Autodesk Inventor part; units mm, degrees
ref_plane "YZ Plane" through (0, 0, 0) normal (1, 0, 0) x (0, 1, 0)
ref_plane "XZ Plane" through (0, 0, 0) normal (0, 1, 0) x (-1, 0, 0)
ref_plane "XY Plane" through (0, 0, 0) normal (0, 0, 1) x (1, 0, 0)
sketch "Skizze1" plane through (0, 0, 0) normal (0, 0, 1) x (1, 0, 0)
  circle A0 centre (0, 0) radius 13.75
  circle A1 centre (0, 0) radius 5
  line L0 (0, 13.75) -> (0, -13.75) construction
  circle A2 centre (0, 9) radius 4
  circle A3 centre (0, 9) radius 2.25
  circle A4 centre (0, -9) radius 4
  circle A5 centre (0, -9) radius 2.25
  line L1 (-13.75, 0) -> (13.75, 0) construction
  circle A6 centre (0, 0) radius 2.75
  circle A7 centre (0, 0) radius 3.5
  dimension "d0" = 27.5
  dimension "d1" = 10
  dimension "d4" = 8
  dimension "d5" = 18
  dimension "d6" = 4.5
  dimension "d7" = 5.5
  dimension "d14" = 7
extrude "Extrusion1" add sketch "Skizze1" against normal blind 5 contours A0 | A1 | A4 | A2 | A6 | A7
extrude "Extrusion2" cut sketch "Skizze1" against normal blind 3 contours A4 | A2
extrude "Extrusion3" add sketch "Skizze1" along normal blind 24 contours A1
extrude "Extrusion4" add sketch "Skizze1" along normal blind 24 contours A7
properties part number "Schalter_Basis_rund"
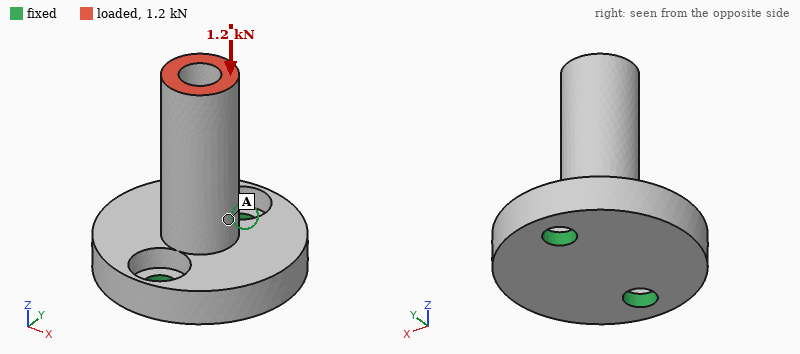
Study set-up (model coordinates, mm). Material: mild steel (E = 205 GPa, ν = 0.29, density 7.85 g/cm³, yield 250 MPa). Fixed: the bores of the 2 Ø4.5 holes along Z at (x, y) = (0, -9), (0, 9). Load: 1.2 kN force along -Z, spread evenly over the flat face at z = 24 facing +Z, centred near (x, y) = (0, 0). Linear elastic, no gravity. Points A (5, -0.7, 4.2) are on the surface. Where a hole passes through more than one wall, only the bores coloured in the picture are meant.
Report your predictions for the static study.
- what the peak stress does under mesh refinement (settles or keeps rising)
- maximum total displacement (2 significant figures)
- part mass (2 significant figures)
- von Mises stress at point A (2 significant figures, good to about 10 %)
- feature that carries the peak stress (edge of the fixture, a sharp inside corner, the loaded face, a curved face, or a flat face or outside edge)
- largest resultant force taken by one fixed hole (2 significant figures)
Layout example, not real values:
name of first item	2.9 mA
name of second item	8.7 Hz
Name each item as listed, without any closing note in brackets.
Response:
what the peak stress does under mesh refinement	keeps rising
maximum total displacement	4.7 µm
part mass	31 g
von Mises stress at point A	19 MPa
feature that carries the peak stress	edge of the fixture
largest resultant force taken by one fixed hole	660 N
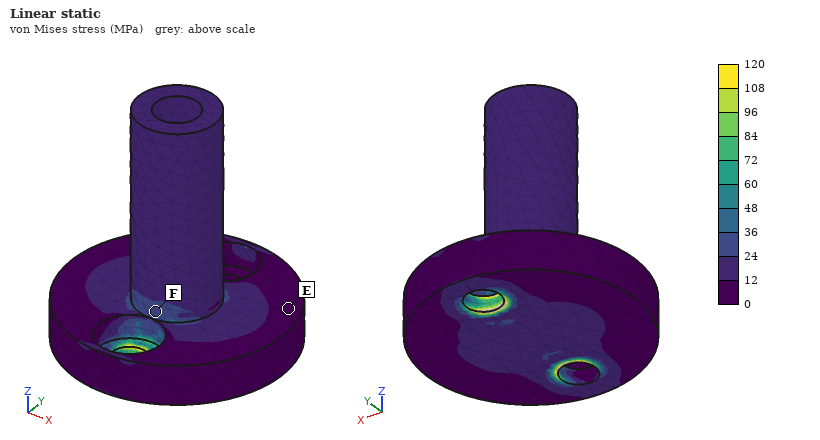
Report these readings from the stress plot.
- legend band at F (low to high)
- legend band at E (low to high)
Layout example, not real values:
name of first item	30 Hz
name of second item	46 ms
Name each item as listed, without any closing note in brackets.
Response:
legend band at F	24 to 36 MPa
legend band at E	0 to 12 MPa
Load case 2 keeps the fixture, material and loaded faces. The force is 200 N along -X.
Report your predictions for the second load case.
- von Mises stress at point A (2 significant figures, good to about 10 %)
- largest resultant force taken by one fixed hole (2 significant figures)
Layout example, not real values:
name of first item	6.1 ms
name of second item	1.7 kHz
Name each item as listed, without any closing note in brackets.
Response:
von Mises stress at point A	42 MPa
largest resultant force taken by one fixed hole	100 N
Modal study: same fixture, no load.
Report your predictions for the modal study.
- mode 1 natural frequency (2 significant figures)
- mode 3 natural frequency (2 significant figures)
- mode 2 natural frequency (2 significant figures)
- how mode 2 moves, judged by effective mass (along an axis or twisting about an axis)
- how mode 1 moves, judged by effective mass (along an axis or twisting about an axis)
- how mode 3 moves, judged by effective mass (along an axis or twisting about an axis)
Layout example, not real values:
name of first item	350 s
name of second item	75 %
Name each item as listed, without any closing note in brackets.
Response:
mode 1 natural frequency	5600 Hz
mode 3 natural frequency	20 kHz
mode 2 natural frequency	9300 Hz
how mode 2 moves, judged by effective mass	along Y
how mode 1 moves, judged by effective mass	along X
how mode 3 moves, judged by effective mass	along Z
